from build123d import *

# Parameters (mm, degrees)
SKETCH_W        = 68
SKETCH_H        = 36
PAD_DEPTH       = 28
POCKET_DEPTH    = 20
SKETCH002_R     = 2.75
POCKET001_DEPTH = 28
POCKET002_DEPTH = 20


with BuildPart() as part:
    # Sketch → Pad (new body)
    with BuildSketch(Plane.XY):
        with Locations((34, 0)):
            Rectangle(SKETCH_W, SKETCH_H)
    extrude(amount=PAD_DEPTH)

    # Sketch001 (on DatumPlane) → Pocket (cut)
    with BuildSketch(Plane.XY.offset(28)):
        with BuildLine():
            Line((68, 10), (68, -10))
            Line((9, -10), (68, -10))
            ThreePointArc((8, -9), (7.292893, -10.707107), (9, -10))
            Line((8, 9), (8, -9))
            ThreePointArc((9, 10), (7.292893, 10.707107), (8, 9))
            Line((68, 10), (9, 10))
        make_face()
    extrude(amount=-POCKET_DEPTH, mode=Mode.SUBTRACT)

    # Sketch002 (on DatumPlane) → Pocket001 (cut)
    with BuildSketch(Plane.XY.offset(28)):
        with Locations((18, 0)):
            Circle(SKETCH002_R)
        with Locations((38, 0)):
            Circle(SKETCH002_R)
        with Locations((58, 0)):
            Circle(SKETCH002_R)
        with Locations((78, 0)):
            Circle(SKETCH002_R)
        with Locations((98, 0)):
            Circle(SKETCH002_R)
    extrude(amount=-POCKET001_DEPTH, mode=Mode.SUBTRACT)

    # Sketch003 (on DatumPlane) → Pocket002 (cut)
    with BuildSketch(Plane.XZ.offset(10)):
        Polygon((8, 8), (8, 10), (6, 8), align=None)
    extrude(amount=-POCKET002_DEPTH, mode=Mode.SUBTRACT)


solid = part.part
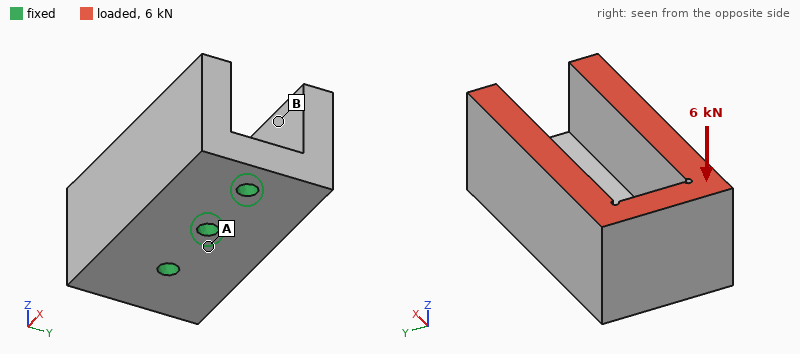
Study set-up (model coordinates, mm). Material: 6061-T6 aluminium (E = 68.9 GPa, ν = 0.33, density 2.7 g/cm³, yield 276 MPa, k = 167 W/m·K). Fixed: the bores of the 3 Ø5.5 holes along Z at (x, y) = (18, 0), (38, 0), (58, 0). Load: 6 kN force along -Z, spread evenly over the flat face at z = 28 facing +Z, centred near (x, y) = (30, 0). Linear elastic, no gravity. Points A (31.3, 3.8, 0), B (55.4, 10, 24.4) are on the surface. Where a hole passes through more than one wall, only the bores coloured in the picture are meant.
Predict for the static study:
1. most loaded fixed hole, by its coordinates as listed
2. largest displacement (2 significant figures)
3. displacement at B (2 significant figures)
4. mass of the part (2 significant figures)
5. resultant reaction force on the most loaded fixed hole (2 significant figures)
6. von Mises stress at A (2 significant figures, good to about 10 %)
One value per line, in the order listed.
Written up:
(18, 0)
25 µm
18 µm
120 g
3.2 kN
22 MPa
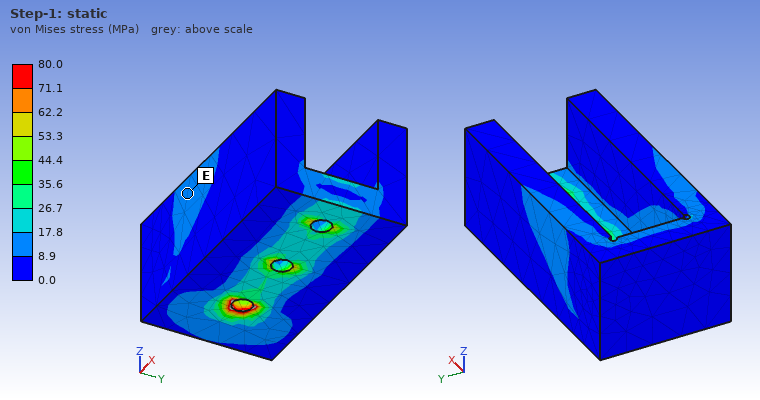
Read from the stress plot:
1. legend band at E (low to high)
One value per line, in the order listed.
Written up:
8.9 to 17.8 MPa
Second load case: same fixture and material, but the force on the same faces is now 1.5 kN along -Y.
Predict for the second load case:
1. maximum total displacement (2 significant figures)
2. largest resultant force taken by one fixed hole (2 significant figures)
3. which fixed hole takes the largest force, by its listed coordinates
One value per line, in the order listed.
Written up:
41 µm
840 N
(18, 0)
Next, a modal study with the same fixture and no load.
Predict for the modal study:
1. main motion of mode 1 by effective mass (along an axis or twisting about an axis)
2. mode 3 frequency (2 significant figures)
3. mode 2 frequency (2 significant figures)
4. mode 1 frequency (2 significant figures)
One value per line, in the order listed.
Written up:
along Y
8300 Hz
7400 Hz
5400 Hz
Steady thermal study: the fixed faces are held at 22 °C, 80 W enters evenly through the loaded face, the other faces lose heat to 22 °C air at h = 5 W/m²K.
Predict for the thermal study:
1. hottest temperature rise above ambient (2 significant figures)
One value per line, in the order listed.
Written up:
17 K
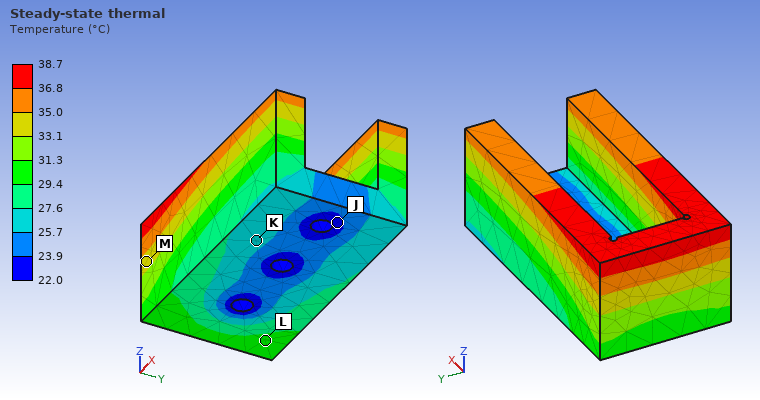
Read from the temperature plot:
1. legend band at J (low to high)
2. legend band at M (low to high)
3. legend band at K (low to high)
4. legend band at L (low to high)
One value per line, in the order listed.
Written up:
22.0 to 23.9 °C
33.1 to 35.0 °C
25.7 to 27.6 °C
29.4 to 31.3 °C
